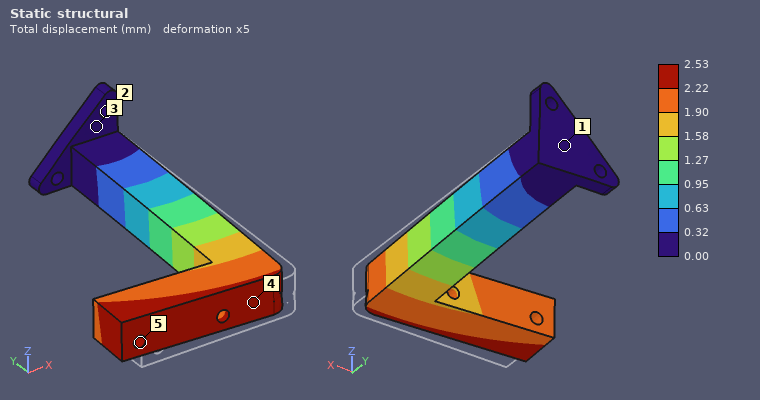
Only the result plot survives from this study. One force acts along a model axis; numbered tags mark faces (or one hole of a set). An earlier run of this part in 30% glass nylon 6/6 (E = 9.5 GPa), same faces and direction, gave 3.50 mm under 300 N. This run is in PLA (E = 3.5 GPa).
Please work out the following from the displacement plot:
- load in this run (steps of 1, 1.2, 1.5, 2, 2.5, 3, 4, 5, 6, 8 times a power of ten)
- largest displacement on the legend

80 N
2.53 mm
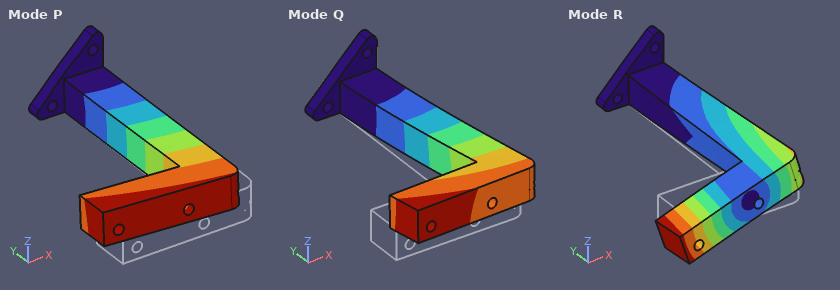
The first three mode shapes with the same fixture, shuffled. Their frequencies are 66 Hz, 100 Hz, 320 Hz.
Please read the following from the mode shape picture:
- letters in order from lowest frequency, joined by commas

P, Q, R
